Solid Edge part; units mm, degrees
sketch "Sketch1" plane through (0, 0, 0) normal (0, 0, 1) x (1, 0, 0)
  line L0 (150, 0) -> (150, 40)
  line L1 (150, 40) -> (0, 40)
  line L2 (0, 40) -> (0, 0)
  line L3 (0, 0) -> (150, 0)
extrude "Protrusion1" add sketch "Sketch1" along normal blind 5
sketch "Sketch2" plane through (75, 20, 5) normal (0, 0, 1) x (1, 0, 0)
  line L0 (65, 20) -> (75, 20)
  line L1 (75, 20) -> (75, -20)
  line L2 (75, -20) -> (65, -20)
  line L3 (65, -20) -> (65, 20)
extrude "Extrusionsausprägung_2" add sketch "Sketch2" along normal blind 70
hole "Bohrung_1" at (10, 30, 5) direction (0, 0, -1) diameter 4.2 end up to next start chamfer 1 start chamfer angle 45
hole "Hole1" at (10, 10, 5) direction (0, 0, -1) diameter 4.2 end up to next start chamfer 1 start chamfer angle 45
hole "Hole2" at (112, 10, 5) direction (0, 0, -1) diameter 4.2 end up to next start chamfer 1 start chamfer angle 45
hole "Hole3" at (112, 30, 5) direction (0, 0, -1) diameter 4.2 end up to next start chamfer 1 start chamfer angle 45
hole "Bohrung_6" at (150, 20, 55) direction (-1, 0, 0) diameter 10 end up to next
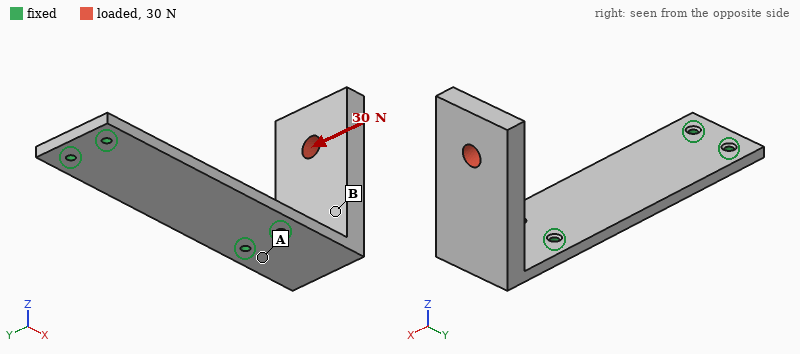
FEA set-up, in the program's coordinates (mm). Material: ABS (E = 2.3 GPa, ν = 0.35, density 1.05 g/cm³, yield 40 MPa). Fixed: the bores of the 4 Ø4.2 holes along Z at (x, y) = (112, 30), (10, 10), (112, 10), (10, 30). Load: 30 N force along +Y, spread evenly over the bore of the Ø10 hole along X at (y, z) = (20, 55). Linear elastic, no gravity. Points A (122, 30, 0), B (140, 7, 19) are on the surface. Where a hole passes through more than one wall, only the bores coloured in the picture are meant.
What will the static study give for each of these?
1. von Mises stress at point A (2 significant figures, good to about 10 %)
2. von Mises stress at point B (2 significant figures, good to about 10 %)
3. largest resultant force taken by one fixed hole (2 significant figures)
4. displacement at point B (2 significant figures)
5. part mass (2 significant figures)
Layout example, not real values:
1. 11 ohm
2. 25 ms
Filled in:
1. 5.0 MPa
2. 0.92 MPa
3. 77 N
4. 0.42 mm
5. 60 g
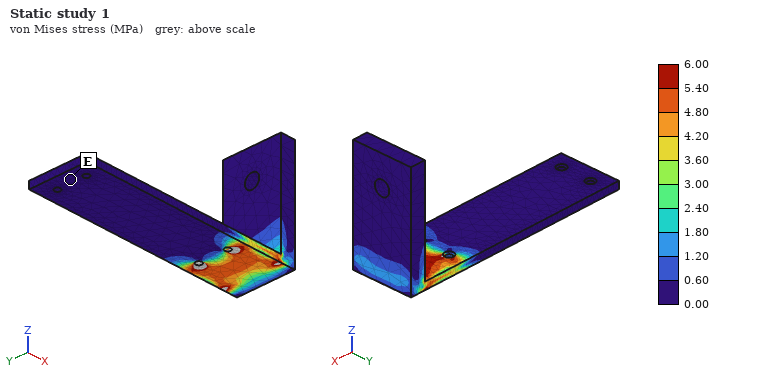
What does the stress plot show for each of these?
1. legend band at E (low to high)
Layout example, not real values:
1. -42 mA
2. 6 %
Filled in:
1. 0.00 to 0.60 MPa
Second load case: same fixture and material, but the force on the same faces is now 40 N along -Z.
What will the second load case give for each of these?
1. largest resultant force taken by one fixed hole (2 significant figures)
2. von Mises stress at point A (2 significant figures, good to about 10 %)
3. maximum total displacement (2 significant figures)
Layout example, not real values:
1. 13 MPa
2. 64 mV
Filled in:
1. 21 N
2. 5.0 MPa
3. 1.8 mm
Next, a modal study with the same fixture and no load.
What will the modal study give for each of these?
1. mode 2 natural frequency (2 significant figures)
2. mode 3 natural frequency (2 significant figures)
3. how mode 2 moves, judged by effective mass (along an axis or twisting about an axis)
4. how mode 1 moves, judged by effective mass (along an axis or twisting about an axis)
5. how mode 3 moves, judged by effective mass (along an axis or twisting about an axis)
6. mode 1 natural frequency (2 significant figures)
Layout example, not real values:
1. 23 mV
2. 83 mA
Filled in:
1. 190 Hz
2. 530 Hz
3. along Y
4. along X
5. along Z
6. 110 Hz
